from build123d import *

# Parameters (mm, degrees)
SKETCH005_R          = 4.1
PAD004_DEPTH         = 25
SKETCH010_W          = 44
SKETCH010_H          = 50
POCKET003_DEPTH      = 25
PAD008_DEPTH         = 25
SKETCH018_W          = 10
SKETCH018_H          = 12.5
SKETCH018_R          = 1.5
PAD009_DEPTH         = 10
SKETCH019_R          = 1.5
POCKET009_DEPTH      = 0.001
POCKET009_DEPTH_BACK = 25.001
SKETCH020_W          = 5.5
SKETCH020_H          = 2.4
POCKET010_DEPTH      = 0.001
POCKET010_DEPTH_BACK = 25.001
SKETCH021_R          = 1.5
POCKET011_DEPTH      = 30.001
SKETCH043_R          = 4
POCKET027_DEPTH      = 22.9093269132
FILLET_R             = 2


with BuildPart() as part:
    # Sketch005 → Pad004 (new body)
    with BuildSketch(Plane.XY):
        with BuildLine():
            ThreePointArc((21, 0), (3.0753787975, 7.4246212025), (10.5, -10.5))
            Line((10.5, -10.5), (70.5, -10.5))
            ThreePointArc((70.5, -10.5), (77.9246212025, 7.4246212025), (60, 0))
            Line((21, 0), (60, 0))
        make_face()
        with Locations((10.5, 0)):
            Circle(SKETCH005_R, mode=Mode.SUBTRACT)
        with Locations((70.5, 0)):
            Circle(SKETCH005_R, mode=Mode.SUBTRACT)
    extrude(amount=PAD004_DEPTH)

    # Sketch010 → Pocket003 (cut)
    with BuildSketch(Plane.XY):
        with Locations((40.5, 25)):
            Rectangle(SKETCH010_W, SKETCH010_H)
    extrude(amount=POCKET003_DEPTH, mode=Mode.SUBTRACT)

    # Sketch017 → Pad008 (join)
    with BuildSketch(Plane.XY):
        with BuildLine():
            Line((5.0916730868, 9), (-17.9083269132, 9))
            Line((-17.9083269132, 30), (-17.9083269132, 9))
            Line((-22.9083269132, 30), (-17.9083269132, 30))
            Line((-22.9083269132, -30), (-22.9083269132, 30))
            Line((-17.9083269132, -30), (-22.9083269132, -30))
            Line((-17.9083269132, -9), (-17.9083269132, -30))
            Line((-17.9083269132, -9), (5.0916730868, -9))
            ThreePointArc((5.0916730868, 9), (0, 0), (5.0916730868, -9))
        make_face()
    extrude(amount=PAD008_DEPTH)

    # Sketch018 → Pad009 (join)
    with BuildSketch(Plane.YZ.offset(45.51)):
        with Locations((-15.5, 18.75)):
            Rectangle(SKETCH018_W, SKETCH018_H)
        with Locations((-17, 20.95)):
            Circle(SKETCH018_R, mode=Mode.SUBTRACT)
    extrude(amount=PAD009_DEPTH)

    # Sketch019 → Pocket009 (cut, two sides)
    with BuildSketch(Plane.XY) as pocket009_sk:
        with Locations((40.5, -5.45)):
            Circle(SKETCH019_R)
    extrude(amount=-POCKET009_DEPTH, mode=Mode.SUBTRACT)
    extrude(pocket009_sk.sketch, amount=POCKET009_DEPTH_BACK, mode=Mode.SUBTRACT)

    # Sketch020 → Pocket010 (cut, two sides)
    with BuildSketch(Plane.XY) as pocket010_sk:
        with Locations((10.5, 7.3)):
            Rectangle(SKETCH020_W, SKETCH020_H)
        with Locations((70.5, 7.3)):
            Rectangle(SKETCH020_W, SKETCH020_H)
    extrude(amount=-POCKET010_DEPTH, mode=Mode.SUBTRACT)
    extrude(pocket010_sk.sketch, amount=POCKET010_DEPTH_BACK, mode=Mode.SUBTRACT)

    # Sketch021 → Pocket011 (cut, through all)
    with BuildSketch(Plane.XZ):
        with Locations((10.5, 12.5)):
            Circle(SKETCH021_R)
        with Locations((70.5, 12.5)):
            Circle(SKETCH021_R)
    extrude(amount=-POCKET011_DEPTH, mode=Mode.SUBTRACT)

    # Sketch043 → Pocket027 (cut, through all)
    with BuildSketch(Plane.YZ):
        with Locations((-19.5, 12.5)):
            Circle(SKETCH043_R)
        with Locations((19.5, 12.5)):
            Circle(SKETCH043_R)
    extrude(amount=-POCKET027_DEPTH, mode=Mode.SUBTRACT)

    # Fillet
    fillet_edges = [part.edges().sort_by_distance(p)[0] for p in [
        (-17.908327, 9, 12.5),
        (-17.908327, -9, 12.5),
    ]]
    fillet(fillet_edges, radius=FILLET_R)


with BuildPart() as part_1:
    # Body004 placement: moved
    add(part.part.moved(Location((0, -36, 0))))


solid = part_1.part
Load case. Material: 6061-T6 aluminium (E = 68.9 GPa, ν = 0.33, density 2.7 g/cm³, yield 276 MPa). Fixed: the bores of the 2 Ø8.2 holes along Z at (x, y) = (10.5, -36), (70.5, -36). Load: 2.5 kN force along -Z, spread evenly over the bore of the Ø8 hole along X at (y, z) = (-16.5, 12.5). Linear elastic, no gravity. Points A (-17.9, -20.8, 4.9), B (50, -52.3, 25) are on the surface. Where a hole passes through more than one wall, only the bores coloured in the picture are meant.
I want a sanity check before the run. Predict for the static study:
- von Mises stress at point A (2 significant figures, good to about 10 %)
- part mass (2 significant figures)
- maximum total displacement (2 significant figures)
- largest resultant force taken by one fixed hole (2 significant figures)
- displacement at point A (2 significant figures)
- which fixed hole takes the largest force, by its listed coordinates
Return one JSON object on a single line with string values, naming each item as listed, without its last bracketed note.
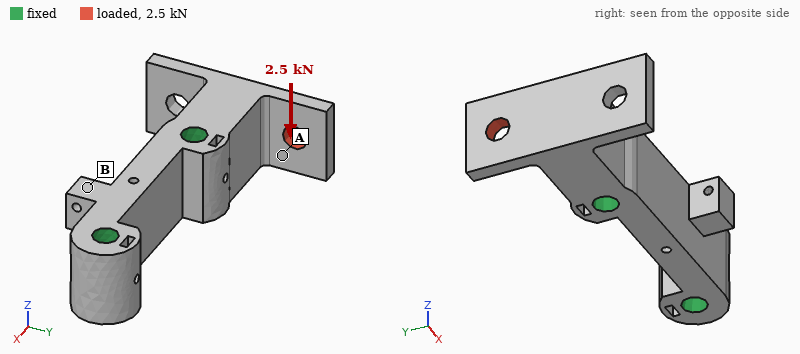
{"von Mises stress at point A": "45 MPa", "part mass": "110 g", "maximum total displacement": "0.11 mm", "largest resultant force taken by one fixed hole": "2.6 kN", "displacement at point A": "0.059 mm", "which fixed hole takes the largest force, by its listed coordinates": "(10.5, -36)"}
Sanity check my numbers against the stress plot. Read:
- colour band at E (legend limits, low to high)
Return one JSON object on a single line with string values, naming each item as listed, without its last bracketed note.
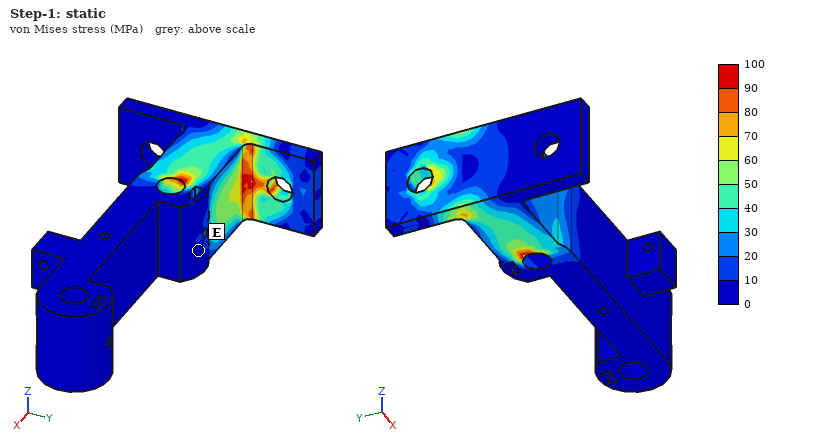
{"colour band at E": "0 to 10 MPa"}
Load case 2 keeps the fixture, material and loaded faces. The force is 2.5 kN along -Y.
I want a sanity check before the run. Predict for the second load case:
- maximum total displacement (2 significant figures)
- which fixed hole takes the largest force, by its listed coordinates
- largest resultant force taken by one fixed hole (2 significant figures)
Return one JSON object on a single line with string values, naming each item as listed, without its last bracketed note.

{"maximum total displacement": "82 µm", "which fixed hole takes the largest force, by its listed coordinates": "(10.5, -36)", "largest resultant force taken by one fixed hole": "2.7 kN"}
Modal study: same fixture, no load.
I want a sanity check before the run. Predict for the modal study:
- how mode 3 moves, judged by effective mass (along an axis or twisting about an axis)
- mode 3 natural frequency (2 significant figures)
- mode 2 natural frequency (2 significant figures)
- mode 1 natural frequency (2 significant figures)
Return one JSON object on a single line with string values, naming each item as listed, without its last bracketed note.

{"how mode 3 moves, judged by effective mass": "twisting about X", "mode 3 natural frequency": "8800 Hz", "mode 2 natural frequency": "7400 Hz", "mode 1 natural frequency": "5600 Hz"}
